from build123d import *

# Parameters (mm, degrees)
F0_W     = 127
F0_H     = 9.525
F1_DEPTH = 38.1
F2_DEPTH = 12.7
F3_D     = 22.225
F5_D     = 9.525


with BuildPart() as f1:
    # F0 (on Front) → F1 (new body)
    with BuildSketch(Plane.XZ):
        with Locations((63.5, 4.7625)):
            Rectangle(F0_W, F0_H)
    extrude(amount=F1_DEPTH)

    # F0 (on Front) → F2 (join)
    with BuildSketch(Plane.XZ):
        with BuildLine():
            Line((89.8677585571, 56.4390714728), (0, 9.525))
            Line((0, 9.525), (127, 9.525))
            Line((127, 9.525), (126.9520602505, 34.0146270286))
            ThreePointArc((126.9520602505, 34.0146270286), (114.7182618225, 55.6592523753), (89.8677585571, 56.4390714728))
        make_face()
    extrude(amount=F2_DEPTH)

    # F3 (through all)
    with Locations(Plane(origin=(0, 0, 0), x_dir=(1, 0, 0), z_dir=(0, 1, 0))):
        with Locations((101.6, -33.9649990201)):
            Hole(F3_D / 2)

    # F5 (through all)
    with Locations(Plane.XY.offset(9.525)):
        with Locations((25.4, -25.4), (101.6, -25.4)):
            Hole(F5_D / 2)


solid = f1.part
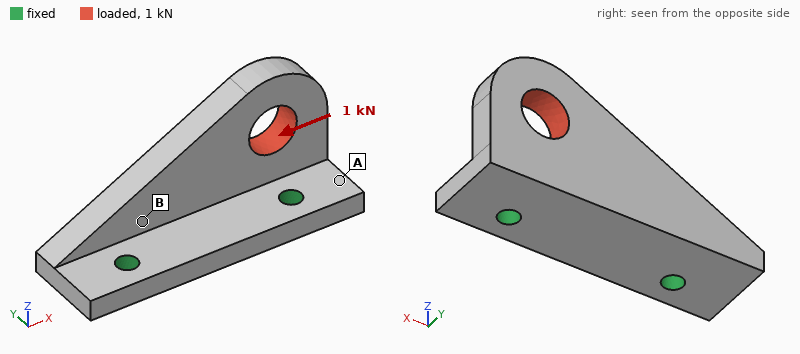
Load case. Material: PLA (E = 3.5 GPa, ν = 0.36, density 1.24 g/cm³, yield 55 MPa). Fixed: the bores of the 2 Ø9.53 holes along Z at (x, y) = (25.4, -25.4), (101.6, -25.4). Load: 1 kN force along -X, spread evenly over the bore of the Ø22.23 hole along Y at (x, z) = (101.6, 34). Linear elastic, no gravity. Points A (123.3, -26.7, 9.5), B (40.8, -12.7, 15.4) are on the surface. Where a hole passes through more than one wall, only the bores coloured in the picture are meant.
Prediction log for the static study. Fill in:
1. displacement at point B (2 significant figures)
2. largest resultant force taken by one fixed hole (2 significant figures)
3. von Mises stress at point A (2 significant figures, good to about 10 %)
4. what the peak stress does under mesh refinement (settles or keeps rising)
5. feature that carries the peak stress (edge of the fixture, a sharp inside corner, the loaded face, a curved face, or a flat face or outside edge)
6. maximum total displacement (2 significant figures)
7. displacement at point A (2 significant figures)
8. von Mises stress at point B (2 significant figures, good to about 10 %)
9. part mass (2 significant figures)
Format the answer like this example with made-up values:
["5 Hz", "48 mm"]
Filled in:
["0.048 mm", "650 N", "1.5 MPa", "keeps rising", "edge of the fixture", "0.19 mm", "0.033 mm", "4.0 MPa", "110 g"]
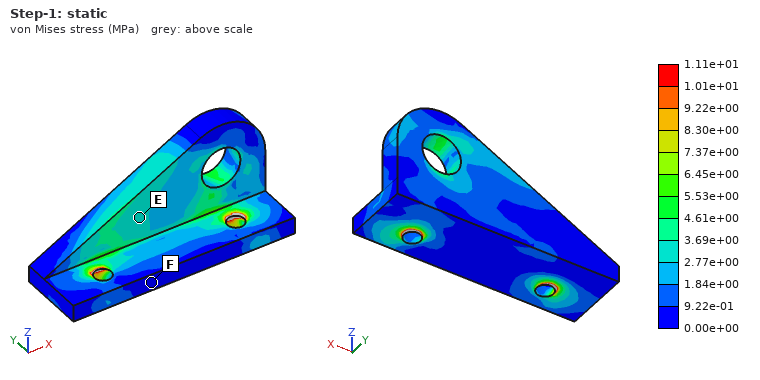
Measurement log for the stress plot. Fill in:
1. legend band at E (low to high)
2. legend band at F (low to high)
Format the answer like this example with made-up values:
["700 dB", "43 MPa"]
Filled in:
["2.77e+00 to 3.69e+00 MPa", "0.00e+00 to 9.22e-01 MPa"]
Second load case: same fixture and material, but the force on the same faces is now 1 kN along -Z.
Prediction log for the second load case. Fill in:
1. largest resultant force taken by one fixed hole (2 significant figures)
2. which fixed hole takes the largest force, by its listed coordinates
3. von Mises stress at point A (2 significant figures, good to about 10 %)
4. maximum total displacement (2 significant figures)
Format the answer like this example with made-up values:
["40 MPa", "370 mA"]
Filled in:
["970 N", "(101.6, -25.4)", "4.5 MPa", "0.61 mm"]
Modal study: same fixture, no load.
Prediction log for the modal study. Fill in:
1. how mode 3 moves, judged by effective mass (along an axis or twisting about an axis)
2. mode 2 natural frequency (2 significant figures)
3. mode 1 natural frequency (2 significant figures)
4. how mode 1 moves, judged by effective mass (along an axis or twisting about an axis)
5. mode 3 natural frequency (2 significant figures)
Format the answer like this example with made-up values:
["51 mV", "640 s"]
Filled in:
["along Z", "1700 Hz", "770 Hz", "along Y", "2200 Hz"]
